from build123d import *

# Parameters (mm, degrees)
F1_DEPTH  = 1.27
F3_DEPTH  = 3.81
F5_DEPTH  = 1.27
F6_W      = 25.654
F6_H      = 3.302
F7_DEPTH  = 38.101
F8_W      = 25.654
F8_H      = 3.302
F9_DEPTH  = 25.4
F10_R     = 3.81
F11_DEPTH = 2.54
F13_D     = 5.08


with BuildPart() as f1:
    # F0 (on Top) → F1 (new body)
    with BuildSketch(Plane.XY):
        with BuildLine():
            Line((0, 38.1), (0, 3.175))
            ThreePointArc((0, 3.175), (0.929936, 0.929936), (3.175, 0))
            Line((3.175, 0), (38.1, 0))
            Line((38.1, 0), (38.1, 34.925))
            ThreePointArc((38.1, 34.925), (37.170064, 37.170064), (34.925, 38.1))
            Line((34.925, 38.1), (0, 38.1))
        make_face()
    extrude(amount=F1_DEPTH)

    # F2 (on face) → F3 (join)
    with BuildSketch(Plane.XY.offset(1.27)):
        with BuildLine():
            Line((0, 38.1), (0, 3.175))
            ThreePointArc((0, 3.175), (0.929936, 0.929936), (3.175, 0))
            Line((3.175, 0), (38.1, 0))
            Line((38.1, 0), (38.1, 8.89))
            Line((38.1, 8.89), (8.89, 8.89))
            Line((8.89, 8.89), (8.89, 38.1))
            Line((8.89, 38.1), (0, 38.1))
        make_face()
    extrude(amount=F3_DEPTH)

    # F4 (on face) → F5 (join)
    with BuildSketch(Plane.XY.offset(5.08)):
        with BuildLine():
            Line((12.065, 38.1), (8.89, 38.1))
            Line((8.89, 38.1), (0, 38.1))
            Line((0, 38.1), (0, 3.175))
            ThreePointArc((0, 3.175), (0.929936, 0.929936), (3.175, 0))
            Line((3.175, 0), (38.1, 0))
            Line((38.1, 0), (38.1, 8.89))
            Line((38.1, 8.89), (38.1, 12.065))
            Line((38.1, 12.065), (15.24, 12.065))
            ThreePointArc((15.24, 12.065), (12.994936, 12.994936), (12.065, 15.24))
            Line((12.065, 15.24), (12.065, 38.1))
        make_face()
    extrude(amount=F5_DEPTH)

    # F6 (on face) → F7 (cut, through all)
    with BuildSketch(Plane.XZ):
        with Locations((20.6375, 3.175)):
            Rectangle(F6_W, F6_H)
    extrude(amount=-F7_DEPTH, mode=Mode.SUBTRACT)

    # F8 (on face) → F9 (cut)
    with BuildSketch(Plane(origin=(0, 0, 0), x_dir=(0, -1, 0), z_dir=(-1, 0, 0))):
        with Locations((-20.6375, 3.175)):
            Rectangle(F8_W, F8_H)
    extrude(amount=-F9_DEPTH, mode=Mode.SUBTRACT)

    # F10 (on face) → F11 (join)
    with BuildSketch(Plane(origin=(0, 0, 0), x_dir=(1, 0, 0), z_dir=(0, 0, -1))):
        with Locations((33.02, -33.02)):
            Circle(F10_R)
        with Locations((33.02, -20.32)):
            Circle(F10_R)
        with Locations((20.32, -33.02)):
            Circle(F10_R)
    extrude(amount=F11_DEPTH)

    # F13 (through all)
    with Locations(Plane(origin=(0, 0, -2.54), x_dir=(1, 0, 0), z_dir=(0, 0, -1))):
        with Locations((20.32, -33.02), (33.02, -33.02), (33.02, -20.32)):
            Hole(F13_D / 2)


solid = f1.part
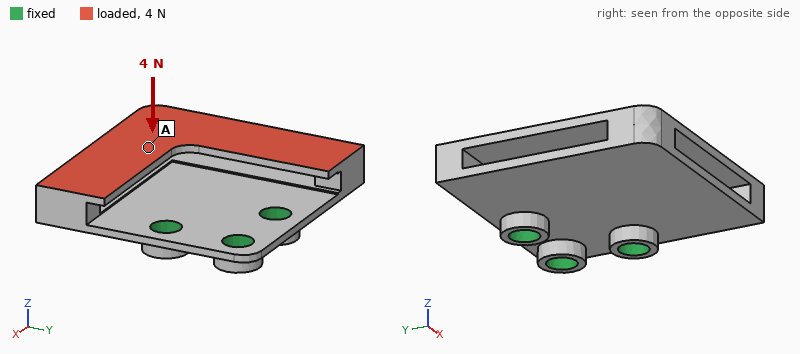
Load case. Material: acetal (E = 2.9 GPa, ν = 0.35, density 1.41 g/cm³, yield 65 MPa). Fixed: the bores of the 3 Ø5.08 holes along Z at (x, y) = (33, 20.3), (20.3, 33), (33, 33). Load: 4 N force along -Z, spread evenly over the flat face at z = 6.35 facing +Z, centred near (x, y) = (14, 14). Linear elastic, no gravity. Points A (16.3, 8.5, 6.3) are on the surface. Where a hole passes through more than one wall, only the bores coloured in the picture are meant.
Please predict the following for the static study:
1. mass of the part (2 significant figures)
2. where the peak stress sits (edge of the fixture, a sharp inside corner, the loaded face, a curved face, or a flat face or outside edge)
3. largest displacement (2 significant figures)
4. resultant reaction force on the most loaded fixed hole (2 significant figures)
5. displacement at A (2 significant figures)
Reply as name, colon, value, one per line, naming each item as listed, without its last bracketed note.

mass of the part: 5.2 g
where the peak stress sits: a flat face or outside edge
largest displacement: 0.60 mm
resultant reaction force on the most loaded fixed hole: 2.3 N
displacement at A: 0.32 mm
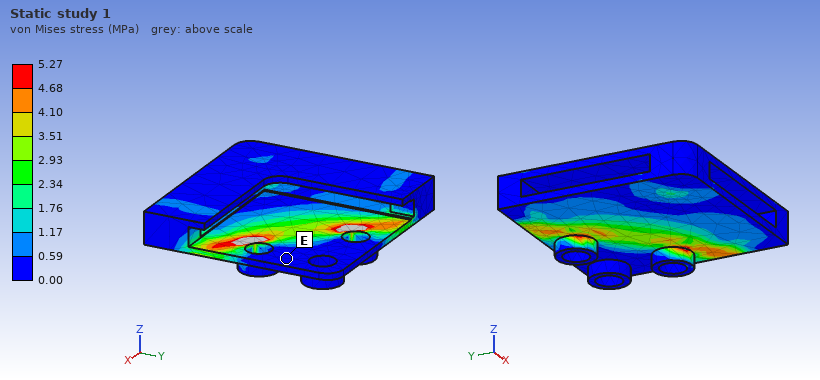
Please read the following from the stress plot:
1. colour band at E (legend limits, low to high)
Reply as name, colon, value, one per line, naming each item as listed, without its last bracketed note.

colour band at E: 0.00 to 0.59 MPa
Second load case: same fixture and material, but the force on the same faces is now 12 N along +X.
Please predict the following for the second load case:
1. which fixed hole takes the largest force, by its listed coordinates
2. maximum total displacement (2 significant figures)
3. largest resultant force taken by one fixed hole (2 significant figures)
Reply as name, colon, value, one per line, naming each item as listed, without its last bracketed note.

which fixed hole takes the largest force, by its listed coordinates: (33, 20.3)
maximum total displacement: 0.56 mm
largest resultant force taken by one fixed hole: 11 N
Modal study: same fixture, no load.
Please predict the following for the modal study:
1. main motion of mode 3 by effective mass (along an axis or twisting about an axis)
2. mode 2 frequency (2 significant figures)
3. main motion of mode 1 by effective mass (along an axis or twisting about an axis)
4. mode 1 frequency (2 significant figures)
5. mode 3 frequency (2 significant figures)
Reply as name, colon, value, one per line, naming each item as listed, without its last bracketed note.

main motion of mode 3 by effective mass: along Z
mode 2 frequency: 670 Hz
main motion of mode 1 by effective mass: along Z
mode 1 frequency: 260 Hz
mode 3 frequency: 1300 Hz
